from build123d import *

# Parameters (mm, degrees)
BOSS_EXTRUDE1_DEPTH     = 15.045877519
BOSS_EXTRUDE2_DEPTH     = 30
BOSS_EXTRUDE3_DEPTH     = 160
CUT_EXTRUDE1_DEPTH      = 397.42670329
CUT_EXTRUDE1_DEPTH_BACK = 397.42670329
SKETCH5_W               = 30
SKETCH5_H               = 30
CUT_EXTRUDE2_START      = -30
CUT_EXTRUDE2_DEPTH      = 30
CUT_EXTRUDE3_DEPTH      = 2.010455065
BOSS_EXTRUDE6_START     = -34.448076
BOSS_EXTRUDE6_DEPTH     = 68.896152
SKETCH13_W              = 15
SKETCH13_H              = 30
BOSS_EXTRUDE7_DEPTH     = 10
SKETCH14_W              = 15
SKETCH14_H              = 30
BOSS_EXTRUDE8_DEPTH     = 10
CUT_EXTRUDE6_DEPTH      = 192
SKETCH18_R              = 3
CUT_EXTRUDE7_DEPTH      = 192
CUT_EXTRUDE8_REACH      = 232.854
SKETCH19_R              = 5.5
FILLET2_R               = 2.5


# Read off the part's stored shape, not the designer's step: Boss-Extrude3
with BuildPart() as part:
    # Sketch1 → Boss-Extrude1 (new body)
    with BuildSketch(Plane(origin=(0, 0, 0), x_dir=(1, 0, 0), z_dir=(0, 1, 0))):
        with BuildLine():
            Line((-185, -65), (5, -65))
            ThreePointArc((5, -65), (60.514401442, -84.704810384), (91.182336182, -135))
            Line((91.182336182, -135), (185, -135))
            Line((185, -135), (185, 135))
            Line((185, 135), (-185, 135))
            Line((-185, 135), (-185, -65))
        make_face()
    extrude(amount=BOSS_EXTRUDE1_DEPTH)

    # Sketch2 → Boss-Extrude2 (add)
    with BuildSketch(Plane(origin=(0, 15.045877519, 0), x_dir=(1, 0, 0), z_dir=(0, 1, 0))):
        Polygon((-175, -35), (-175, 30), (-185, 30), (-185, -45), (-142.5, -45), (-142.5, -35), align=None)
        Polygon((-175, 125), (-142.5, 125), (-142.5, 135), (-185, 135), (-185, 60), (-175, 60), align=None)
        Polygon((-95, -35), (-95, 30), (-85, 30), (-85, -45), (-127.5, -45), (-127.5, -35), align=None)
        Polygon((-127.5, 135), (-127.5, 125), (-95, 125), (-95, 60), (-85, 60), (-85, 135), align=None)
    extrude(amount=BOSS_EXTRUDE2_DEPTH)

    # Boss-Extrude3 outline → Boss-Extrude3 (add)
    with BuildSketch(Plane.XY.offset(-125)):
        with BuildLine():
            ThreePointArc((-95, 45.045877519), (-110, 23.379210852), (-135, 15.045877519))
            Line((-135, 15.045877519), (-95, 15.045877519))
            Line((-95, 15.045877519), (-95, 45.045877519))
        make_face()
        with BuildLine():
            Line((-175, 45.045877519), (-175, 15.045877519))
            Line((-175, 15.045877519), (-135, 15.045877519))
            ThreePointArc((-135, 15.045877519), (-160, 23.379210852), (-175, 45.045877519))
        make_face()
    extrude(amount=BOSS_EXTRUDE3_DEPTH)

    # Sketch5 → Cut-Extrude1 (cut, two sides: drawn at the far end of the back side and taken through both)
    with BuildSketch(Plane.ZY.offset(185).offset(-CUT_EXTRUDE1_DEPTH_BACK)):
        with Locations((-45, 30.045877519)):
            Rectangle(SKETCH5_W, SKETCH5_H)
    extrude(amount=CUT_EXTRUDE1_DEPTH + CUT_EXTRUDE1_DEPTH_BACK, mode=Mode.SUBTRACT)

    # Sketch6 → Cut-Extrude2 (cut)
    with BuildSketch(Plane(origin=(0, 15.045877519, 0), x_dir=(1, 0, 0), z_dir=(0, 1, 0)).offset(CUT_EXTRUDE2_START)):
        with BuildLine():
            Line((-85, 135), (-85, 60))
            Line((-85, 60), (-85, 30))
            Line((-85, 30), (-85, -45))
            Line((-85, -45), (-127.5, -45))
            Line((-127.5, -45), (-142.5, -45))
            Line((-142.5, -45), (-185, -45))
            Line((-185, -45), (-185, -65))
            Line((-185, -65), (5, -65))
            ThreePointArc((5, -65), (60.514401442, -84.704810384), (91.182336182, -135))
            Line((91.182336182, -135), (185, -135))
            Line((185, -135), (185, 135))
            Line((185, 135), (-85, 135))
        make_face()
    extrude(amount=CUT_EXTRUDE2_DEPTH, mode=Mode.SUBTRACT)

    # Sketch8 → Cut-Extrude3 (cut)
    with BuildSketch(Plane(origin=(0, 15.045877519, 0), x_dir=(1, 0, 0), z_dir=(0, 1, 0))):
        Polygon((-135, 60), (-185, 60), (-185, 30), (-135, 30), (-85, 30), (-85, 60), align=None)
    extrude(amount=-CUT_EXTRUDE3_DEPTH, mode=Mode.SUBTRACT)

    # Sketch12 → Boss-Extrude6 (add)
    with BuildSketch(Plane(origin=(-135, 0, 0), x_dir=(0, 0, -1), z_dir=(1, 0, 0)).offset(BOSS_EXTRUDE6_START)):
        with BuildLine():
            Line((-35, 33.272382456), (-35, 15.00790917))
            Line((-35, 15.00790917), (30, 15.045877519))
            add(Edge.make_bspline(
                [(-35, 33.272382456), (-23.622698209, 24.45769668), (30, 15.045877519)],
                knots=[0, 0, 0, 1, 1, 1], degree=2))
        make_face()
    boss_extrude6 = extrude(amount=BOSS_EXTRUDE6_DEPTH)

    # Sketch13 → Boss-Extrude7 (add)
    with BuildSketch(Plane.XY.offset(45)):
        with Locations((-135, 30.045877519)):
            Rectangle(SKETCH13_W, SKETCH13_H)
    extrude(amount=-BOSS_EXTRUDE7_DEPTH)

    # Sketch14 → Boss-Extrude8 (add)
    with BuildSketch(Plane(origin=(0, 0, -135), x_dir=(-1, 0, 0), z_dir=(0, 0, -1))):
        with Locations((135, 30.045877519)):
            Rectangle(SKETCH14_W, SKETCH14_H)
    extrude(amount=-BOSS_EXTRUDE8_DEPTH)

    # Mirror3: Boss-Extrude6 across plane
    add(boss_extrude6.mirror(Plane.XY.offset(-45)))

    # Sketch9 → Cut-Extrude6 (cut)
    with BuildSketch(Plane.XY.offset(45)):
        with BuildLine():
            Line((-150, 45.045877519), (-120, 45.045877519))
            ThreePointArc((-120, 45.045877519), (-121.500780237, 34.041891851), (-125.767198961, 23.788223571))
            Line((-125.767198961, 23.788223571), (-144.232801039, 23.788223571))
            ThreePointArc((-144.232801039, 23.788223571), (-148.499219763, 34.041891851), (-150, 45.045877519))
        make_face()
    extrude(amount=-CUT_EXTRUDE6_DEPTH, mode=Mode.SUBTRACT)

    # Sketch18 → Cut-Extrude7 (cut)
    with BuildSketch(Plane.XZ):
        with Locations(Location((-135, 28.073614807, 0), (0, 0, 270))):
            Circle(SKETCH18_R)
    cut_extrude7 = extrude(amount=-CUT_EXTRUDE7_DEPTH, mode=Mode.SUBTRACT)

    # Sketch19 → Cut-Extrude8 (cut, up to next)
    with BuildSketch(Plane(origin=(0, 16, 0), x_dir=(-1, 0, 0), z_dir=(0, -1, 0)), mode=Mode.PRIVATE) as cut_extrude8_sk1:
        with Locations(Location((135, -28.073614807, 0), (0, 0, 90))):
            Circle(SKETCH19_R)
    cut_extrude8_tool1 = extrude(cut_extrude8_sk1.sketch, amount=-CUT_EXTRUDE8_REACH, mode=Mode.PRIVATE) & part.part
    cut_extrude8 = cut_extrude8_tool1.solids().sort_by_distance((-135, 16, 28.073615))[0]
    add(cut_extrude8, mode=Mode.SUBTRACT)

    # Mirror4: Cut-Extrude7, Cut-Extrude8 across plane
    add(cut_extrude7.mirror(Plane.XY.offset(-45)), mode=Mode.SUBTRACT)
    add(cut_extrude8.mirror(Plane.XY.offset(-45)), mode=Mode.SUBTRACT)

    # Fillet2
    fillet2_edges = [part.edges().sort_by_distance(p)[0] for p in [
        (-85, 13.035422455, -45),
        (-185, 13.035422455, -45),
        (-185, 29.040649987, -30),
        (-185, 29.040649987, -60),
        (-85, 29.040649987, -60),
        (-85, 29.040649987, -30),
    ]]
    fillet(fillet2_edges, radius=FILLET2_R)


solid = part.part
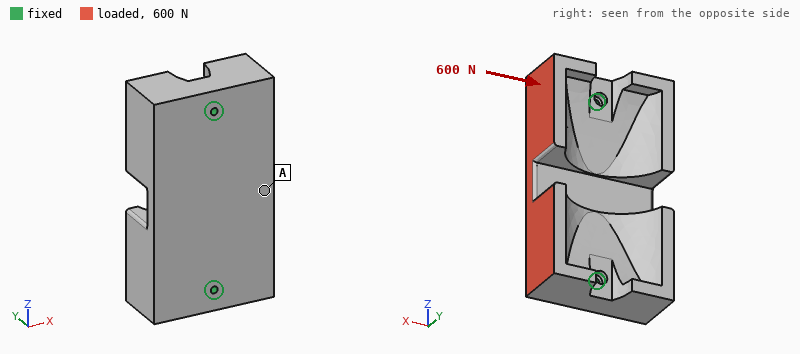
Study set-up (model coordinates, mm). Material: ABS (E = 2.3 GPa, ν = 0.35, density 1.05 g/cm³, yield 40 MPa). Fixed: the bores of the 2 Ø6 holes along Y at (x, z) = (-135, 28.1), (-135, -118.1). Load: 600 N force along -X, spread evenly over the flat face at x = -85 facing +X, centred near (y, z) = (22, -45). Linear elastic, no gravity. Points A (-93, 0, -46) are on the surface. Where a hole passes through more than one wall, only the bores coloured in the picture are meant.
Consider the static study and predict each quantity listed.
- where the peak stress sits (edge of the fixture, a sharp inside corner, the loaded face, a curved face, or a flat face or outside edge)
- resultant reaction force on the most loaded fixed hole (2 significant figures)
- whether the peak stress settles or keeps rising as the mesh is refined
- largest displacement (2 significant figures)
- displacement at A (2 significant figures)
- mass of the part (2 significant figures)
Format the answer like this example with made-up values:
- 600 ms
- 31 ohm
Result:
- edge of the fixture
- 300 N
- keeps rising
- 0.11 mm
- 0.061 mm
- 530 g
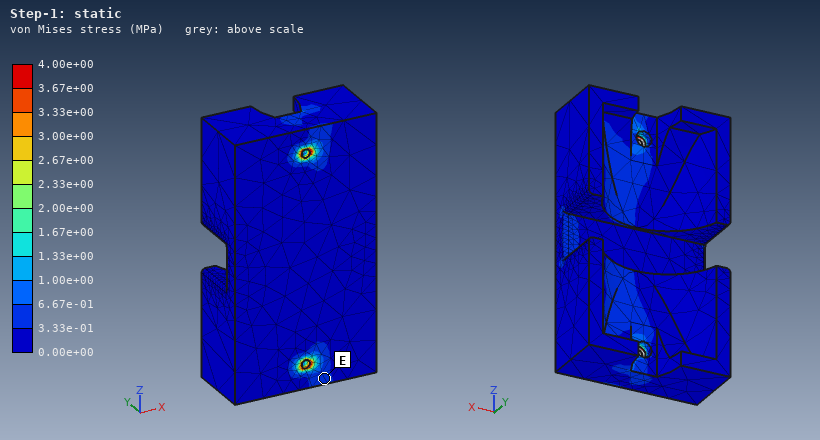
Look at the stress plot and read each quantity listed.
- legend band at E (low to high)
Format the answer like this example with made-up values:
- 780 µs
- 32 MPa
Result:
- 3.33e-01 to 6.67e-01 MPa
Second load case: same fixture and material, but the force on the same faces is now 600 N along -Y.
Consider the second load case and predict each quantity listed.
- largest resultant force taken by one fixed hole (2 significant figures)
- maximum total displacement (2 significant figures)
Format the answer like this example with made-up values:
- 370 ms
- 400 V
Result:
- 300 N
- 0.46 mm
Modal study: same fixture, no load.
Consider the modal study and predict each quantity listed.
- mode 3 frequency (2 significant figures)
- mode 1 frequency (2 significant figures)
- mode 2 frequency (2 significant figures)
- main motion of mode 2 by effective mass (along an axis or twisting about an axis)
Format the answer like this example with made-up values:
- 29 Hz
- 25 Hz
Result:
- 840 Hz
- 480 Hz
- 600 Hz
- along Y
